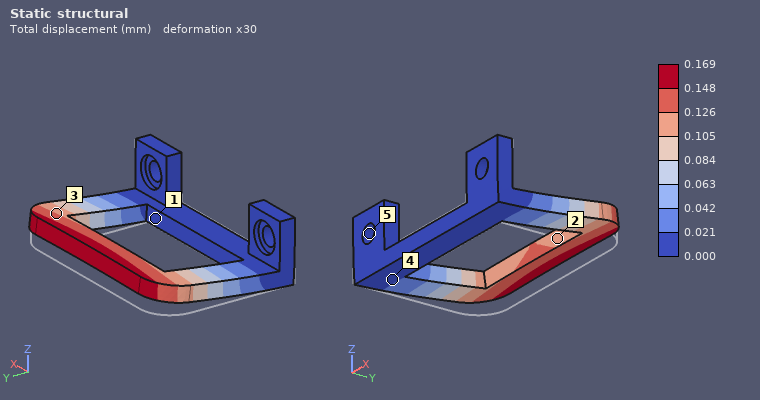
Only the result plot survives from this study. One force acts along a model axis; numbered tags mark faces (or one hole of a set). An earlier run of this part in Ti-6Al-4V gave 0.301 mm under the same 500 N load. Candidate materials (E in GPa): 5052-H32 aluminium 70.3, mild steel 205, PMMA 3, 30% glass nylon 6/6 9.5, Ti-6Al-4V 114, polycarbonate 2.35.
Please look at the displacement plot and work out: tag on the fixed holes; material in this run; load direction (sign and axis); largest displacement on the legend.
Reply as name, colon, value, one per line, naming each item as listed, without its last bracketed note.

tag on the fixed holes: 5
material in this run: mild steel
load direction: +Z
largest displacement on the legend: 0.169 mm
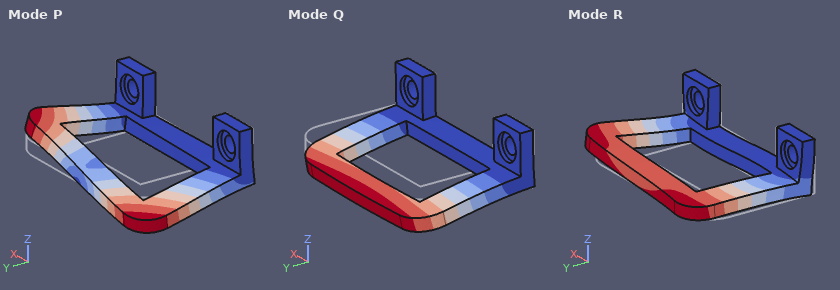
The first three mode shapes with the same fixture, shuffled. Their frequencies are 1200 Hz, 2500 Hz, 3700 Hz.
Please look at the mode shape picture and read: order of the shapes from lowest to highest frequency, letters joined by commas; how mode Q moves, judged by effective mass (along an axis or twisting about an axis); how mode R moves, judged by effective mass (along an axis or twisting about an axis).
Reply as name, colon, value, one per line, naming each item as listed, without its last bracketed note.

order of the shapes from lowest to highest frequency, letters joined by commas: Q, P, R
how mode Q moves, judged by effective mass: along Z
how mode R moves, judged by effective mass: along X
